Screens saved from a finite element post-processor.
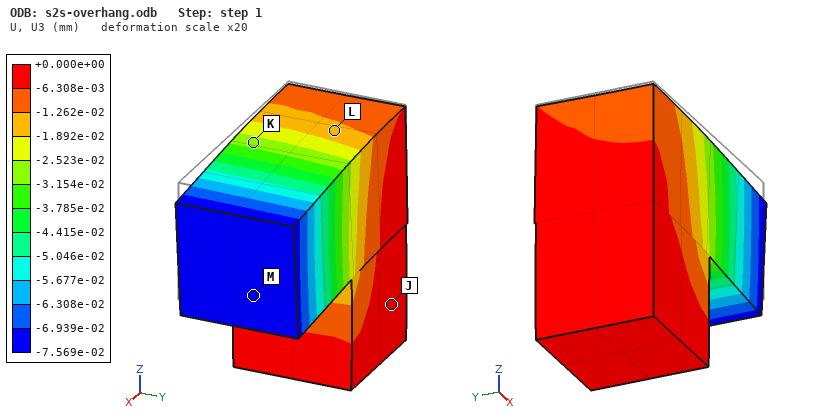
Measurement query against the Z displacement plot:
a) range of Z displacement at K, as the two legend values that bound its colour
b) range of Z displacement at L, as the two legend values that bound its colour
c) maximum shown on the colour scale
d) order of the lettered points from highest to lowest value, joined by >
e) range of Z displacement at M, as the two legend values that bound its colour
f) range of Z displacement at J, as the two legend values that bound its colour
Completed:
-3.154e-02 to -2.523e-02 mm
-1.892e-02 to -1.262e-02 mm
+0.000e+00 mm
J > L > K > M
-7.569e-02 to -6.939e-02 mm
-6.308e-03 to +0.000e+00 mm
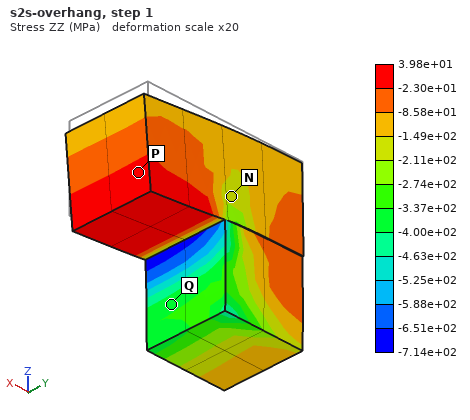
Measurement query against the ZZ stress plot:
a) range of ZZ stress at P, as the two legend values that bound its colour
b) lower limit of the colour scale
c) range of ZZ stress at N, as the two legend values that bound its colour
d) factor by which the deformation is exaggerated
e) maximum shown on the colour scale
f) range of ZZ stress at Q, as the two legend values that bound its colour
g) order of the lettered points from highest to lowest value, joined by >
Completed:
-2.30e+01 to 3.98e+01 MPa
-7.14e+02 MPa
-2.11e+02 to -1.49e+02 MPa
20
3.98e+01 MPa
-4.00e+02 to -3.37e+02 MPa
P > N > Q
